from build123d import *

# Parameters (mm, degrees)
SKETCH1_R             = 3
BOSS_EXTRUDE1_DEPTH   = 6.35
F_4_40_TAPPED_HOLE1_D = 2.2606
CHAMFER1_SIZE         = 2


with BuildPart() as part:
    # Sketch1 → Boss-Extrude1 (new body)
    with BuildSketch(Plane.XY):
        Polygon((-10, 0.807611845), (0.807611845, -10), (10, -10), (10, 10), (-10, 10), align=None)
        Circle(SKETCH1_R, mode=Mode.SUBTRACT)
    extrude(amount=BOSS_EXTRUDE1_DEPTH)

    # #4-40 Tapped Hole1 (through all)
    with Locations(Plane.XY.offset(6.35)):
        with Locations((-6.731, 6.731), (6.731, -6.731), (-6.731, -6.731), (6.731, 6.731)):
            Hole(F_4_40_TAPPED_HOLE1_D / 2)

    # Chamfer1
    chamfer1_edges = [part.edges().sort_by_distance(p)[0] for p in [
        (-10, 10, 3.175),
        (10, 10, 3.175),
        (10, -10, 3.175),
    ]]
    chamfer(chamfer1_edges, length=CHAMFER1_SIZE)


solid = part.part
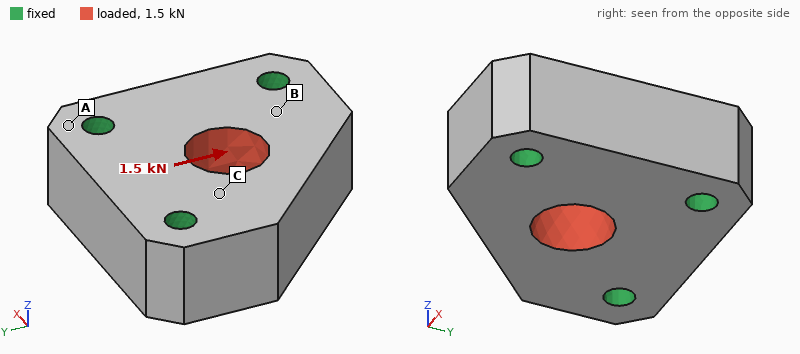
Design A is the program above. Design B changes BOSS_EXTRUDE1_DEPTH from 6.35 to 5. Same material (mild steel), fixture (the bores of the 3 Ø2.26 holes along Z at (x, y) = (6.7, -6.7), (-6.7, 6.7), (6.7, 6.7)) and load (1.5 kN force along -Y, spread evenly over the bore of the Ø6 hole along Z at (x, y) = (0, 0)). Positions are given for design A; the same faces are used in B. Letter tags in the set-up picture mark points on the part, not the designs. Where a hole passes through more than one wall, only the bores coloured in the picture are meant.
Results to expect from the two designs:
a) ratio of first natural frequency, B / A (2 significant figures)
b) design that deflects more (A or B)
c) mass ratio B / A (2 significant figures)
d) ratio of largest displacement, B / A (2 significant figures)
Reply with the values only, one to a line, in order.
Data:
0.88
B
0.79
1.3
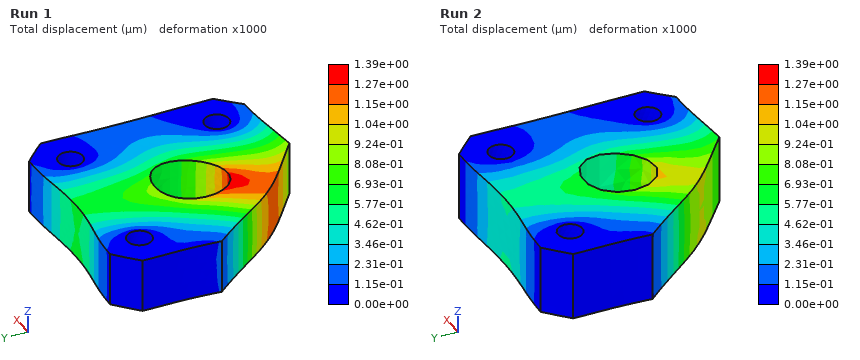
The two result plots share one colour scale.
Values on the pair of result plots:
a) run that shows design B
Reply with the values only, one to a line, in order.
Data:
Run 1
